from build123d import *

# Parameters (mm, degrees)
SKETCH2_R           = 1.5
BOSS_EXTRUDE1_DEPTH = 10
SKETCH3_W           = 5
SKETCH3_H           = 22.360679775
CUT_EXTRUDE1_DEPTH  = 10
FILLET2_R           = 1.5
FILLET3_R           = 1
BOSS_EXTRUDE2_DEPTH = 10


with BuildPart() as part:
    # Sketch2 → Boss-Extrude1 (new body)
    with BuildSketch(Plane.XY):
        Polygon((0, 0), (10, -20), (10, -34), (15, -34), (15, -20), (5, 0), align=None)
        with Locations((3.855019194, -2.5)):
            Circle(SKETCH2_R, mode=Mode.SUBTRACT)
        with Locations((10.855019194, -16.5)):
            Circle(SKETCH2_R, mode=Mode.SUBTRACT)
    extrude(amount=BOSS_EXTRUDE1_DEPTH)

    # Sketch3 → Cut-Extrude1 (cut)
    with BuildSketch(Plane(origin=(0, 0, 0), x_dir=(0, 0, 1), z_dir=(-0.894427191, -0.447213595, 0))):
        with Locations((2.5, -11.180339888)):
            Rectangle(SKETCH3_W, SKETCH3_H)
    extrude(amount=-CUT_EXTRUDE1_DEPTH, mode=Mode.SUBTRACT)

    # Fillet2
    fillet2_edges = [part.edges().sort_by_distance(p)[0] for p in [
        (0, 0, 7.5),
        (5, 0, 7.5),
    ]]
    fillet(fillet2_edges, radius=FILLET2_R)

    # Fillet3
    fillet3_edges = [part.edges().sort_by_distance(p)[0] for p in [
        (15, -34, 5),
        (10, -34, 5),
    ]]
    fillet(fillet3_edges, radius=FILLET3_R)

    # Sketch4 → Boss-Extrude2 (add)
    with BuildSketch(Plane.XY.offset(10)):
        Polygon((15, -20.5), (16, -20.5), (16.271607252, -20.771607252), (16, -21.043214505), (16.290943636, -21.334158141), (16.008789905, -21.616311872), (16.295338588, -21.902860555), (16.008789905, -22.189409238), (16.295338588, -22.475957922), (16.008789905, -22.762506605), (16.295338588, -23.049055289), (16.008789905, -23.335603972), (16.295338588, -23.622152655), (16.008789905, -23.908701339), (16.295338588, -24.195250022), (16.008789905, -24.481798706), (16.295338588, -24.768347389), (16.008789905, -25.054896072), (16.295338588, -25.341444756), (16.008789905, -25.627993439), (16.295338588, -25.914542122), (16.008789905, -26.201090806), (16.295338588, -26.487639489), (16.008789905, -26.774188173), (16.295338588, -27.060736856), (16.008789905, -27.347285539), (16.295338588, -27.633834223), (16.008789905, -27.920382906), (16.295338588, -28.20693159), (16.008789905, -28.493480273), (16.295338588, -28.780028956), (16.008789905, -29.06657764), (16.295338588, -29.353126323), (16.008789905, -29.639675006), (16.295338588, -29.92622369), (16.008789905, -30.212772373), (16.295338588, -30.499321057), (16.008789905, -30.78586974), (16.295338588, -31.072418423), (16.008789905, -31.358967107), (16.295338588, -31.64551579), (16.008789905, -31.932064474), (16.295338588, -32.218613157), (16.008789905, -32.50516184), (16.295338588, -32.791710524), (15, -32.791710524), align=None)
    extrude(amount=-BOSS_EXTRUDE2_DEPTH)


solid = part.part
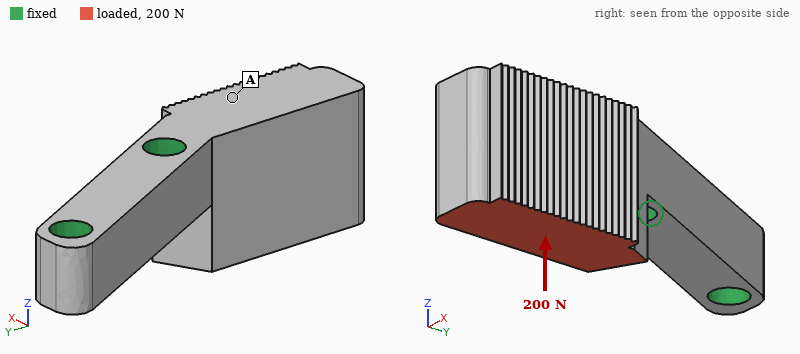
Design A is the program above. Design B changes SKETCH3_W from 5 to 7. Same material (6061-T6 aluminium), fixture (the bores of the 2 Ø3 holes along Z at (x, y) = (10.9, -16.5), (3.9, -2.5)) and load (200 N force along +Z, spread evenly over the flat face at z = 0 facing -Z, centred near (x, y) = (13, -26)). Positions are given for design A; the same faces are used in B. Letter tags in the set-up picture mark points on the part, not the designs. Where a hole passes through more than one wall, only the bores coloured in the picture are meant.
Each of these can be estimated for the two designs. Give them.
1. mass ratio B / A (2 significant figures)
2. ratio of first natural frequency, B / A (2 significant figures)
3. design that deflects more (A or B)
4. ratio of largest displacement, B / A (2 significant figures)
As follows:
0.94
0.88
B
1.7
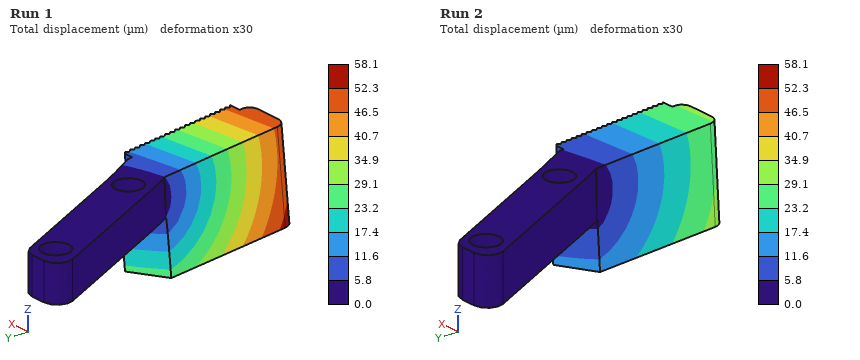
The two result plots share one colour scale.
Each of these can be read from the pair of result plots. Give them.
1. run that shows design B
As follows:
Run 1
